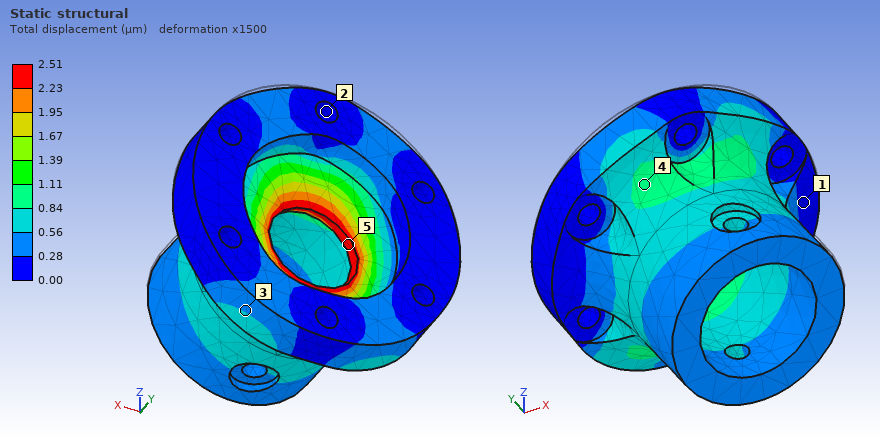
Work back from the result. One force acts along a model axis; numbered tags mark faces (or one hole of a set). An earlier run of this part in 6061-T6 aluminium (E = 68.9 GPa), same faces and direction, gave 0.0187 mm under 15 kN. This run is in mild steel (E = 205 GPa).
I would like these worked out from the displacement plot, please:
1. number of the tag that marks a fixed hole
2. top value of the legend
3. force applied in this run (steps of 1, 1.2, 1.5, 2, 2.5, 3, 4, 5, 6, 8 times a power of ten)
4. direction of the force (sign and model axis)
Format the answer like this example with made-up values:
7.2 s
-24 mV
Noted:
2
2.51 µm
6 kN
-Z
